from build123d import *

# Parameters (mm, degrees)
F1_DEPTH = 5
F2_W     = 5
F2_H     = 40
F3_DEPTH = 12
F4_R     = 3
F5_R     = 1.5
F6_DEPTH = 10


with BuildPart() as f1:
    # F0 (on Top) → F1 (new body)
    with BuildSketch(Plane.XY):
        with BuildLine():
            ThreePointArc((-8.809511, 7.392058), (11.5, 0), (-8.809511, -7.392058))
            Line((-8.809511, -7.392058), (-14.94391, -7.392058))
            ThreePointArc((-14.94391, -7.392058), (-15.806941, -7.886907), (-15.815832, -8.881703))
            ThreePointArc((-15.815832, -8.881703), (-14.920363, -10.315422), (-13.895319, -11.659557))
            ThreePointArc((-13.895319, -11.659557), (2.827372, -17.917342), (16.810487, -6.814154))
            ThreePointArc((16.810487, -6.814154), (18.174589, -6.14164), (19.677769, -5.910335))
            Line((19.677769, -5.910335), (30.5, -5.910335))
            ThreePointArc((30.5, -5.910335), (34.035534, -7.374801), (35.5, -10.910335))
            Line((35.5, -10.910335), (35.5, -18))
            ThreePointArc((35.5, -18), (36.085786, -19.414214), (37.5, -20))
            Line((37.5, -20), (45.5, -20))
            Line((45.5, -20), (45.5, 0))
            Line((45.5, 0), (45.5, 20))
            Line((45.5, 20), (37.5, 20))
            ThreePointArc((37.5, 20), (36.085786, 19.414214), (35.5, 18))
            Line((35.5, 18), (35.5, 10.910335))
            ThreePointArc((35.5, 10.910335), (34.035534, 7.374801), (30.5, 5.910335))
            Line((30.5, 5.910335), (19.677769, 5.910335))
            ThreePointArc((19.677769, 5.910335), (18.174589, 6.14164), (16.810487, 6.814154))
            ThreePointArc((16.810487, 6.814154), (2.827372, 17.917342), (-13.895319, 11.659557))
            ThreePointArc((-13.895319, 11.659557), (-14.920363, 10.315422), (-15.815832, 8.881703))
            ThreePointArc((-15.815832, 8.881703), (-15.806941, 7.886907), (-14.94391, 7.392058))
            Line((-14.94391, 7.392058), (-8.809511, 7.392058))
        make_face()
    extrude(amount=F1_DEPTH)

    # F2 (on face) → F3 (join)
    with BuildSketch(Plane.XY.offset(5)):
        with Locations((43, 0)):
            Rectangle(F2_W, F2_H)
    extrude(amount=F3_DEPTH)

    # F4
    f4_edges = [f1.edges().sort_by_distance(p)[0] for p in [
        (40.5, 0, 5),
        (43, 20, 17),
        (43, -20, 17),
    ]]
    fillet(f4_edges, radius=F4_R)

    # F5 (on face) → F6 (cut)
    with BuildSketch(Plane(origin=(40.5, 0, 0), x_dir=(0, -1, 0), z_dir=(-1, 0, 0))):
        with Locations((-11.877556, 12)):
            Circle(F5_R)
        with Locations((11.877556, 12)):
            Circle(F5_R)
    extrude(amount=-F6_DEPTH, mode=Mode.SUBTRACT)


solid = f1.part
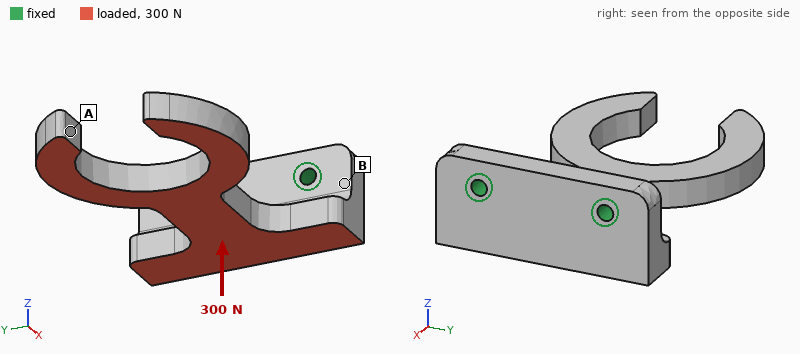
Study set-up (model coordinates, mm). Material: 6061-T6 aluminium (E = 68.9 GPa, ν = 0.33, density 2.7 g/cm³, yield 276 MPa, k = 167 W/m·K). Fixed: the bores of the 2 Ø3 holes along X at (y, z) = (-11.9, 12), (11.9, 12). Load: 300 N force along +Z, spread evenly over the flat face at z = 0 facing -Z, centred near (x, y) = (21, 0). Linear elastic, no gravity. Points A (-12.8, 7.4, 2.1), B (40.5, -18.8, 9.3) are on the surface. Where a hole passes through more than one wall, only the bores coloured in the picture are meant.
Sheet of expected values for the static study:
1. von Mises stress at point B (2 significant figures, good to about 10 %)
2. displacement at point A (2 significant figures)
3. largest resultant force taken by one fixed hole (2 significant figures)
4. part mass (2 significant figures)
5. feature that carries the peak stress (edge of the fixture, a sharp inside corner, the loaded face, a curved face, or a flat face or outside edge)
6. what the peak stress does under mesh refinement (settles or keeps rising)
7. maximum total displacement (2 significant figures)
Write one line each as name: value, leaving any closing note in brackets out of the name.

von Mises stress at point B: 25 MPa
displacement at point A: 0.58 mm
largest resultant force taken by one fixed hole: 170 N
part mass: 22 g
feature that carries the peak stress: edge of the fixture
what the peak stress does under mesh refinement: keeps rising
maximum total displacement: 0.62 mm
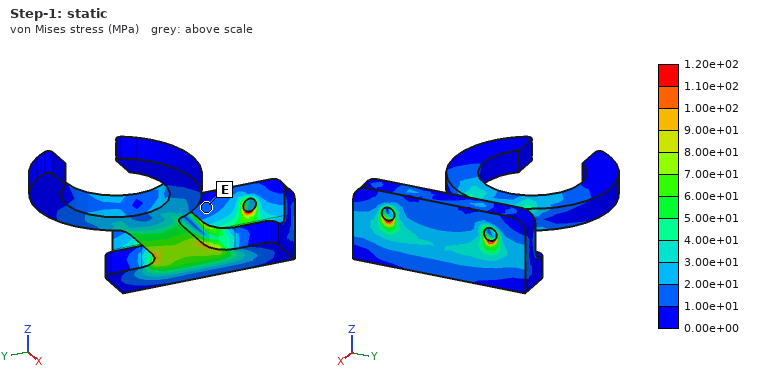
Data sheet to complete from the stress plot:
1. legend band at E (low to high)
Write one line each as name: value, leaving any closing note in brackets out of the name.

legend band at E: 1.00e+01 to 2.00e+01 MPa
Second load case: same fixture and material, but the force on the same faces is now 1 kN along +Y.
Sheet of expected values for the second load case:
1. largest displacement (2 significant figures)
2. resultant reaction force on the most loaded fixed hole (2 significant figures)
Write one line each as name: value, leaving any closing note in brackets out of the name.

largest displacement: 0.43 mm
resultant reaction force on the most loaded fixed hole: 1.1 kN
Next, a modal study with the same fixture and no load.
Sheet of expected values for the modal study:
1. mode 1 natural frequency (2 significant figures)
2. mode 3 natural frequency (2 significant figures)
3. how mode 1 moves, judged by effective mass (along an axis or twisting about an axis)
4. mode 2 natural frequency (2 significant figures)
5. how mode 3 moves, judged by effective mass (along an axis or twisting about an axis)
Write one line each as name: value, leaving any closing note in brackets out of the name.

mode 1 natural frequency: 1100 Hz
mode 3 natural frequency: 2500 Hz
how mode 1 moves, judged by effective mass: along Z
mode 2 natural frequency: 2300 Hz
how mode 3 moves, judged by effective mass: along Y
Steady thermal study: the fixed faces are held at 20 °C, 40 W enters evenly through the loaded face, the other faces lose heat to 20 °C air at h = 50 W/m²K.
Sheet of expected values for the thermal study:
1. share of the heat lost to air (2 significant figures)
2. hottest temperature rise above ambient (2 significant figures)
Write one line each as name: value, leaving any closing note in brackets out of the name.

share of the heat lost to air: 14 %
hottest temperature rise above ambient: 72 K
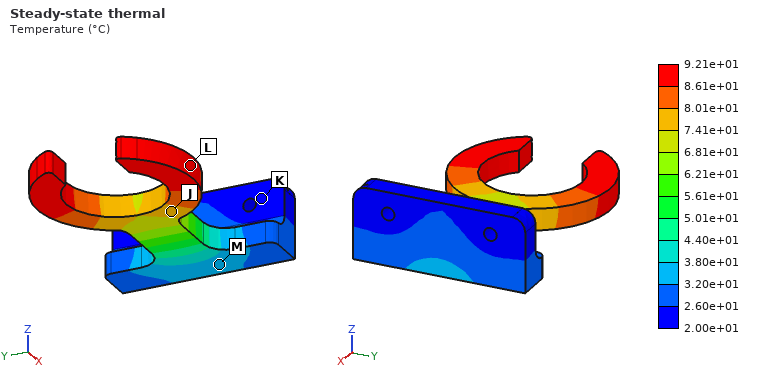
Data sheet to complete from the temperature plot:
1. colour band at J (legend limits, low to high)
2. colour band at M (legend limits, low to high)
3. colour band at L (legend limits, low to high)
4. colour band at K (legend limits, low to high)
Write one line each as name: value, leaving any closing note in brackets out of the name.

colour band at J: 7.41e+01 to 8.01e+01 °C
colour band at M: 3.20e+01 to 3.80e+01 °C
colour band at L: 8.61e+01 to 9.21e+01 °C
colour band at K: 2.00e+01 to 2.60e+01 °C
